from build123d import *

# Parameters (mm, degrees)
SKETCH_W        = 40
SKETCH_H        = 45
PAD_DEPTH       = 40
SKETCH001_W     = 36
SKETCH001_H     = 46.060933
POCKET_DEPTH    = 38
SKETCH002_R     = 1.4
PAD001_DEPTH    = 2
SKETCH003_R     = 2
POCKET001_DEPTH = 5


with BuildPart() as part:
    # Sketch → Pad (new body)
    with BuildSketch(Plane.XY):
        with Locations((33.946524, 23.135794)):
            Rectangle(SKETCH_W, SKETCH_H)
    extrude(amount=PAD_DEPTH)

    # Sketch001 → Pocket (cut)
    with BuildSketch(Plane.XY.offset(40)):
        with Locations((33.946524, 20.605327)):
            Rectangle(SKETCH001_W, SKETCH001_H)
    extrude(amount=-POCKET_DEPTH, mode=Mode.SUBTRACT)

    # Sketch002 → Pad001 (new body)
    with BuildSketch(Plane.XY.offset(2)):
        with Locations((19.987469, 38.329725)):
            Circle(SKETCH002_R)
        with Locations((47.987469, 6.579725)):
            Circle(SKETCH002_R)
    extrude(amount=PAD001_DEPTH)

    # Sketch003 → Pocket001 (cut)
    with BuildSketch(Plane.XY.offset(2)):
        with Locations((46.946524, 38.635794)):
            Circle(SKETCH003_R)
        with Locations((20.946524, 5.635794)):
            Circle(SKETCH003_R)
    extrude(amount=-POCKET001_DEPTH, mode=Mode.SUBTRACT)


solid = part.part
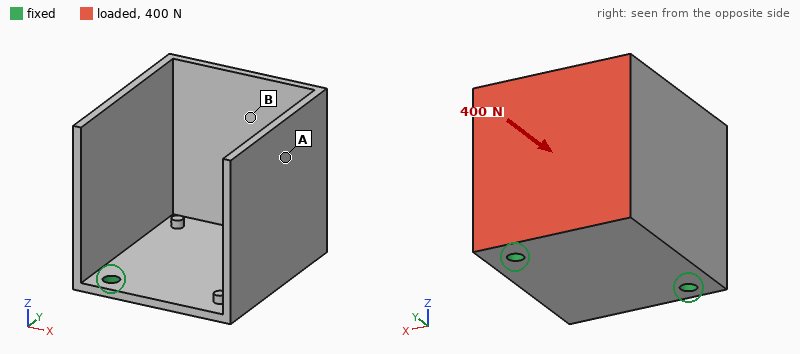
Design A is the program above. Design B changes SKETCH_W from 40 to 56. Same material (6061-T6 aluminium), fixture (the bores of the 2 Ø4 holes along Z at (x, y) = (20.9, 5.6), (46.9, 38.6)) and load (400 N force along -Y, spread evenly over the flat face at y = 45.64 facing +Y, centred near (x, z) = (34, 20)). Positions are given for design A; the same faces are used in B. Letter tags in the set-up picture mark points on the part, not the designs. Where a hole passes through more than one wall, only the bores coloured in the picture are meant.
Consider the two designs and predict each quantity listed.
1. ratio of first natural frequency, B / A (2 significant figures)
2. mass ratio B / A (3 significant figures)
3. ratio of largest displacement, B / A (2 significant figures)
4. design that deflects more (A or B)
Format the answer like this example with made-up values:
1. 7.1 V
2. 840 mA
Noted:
1. 0.55
2. 3.19
3. 0.71
4. A
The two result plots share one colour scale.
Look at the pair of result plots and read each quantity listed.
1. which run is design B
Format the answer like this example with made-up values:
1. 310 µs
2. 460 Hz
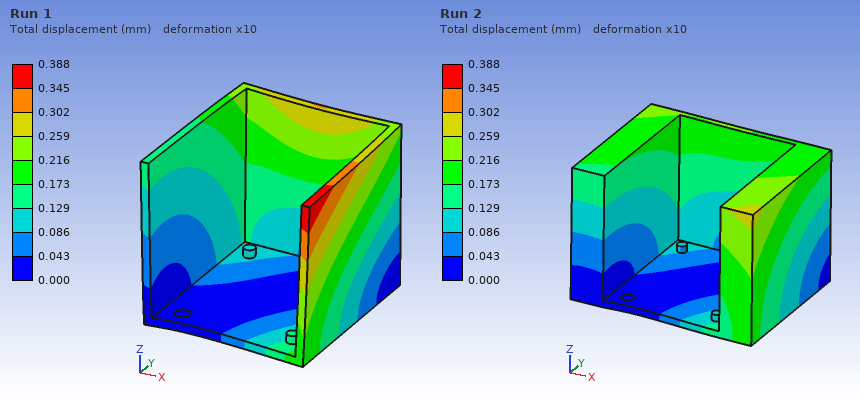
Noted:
1. Run 2
